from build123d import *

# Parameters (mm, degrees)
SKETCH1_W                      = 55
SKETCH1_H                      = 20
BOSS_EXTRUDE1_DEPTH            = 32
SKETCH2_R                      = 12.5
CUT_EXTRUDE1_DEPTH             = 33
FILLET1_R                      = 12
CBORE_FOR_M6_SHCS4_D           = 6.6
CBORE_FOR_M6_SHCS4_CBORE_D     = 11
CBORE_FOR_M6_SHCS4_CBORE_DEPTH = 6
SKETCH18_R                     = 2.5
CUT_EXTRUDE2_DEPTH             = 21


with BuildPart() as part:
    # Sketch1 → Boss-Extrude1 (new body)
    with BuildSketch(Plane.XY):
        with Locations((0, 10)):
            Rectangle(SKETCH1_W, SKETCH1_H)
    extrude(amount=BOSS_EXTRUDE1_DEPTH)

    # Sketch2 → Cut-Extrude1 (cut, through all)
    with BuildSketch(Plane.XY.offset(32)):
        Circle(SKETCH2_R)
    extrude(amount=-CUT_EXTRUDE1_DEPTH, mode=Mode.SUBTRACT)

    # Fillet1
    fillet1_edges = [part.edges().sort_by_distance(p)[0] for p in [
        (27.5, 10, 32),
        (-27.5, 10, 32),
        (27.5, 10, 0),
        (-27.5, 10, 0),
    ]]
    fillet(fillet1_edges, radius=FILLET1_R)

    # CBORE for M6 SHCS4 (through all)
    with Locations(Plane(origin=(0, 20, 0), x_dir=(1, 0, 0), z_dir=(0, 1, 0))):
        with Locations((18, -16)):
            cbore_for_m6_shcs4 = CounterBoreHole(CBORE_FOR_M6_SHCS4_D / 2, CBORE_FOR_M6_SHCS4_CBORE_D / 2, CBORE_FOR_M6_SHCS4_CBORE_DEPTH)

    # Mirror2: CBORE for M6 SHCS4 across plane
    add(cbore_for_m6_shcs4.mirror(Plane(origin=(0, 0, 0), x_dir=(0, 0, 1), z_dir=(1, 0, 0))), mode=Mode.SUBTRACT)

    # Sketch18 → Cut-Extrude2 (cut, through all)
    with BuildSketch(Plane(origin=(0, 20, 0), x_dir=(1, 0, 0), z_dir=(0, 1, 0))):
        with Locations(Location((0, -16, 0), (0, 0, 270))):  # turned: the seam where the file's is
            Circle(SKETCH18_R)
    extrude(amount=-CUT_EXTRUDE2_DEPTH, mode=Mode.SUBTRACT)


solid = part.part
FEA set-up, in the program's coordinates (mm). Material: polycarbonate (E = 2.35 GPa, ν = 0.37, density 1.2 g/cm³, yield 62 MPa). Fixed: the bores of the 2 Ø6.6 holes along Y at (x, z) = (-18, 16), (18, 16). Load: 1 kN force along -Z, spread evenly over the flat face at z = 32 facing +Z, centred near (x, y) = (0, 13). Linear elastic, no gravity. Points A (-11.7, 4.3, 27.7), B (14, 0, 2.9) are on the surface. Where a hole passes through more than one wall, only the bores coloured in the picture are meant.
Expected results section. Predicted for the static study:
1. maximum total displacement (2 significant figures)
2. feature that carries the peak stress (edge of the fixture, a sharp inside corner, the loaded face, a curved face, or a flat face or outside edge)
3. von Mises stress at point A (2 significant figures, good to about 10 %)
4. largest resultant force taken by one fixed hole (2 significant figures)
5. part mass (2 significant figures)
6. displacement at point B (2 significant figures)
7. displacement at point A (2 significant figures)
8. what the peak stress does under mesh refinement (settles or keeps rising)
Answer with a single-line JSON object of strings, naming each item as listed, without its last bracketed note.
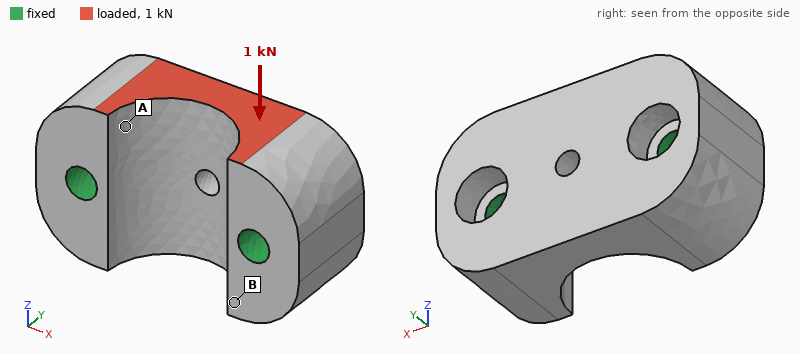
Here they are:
{"maximum total displacement": "71 µm", "feature that carries the peak stress": "edge of the fixture", "von Mises stress at point A": "3.1 MPa", "largest resultant force taken by one fixed hole": "500 N", "part mass": "27 g", "displacement at point B": "14 µm", "displacement at point A": "22 µm", "what the peak stress does under mesh refinement": "keeps rising"}
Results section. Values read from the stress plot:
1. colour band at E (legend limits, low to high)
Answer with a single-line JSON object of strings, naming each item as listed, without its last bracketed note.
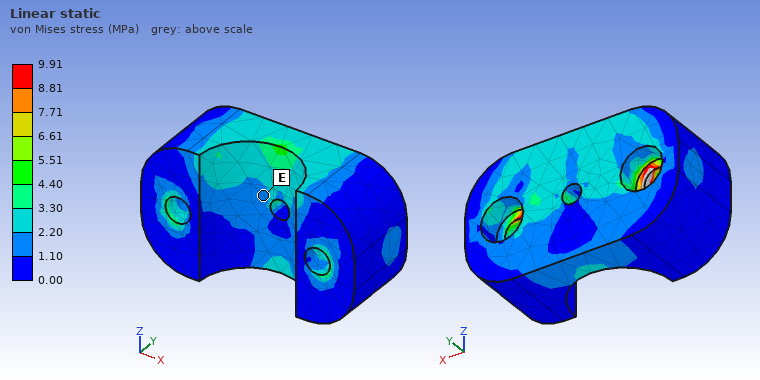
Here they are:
{"colour band at E": "1.10 to 2.20 MPa"}
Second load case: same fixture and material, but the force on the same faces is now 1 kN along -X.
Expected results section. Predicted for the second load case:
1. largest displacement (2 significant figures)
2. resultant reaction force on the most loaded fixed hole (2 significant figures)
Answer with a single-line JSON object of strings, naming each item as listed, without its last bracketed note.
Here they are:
{"largest displacement": "64 µm", "resultant reaction force on the most loaded fixed hole": "600 N"}
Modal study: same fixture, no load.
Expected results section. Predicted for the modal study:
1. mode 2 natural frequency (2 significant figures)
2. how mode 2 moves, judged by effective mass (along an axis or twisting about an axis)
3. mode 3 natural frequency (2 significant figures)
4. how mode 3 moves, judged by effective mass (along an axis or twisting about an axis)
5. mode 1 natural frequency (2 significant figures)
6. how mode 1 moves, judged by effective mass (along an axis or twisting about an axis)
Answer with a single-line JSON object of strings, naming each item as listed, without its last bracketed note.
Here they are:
{"mode 2 natural frequency": "7700 Hz", "how mode 2 moves, judged by effective mass": "twisting about Y", "mode 3 natural frequency": "8100 Hz", "how mode 3 moves, judged by effective mass": "along Y", "mode 1 natural frequency": "5800 Hz", "how mode 1 moves, judged by effective mass": "along Z"}
